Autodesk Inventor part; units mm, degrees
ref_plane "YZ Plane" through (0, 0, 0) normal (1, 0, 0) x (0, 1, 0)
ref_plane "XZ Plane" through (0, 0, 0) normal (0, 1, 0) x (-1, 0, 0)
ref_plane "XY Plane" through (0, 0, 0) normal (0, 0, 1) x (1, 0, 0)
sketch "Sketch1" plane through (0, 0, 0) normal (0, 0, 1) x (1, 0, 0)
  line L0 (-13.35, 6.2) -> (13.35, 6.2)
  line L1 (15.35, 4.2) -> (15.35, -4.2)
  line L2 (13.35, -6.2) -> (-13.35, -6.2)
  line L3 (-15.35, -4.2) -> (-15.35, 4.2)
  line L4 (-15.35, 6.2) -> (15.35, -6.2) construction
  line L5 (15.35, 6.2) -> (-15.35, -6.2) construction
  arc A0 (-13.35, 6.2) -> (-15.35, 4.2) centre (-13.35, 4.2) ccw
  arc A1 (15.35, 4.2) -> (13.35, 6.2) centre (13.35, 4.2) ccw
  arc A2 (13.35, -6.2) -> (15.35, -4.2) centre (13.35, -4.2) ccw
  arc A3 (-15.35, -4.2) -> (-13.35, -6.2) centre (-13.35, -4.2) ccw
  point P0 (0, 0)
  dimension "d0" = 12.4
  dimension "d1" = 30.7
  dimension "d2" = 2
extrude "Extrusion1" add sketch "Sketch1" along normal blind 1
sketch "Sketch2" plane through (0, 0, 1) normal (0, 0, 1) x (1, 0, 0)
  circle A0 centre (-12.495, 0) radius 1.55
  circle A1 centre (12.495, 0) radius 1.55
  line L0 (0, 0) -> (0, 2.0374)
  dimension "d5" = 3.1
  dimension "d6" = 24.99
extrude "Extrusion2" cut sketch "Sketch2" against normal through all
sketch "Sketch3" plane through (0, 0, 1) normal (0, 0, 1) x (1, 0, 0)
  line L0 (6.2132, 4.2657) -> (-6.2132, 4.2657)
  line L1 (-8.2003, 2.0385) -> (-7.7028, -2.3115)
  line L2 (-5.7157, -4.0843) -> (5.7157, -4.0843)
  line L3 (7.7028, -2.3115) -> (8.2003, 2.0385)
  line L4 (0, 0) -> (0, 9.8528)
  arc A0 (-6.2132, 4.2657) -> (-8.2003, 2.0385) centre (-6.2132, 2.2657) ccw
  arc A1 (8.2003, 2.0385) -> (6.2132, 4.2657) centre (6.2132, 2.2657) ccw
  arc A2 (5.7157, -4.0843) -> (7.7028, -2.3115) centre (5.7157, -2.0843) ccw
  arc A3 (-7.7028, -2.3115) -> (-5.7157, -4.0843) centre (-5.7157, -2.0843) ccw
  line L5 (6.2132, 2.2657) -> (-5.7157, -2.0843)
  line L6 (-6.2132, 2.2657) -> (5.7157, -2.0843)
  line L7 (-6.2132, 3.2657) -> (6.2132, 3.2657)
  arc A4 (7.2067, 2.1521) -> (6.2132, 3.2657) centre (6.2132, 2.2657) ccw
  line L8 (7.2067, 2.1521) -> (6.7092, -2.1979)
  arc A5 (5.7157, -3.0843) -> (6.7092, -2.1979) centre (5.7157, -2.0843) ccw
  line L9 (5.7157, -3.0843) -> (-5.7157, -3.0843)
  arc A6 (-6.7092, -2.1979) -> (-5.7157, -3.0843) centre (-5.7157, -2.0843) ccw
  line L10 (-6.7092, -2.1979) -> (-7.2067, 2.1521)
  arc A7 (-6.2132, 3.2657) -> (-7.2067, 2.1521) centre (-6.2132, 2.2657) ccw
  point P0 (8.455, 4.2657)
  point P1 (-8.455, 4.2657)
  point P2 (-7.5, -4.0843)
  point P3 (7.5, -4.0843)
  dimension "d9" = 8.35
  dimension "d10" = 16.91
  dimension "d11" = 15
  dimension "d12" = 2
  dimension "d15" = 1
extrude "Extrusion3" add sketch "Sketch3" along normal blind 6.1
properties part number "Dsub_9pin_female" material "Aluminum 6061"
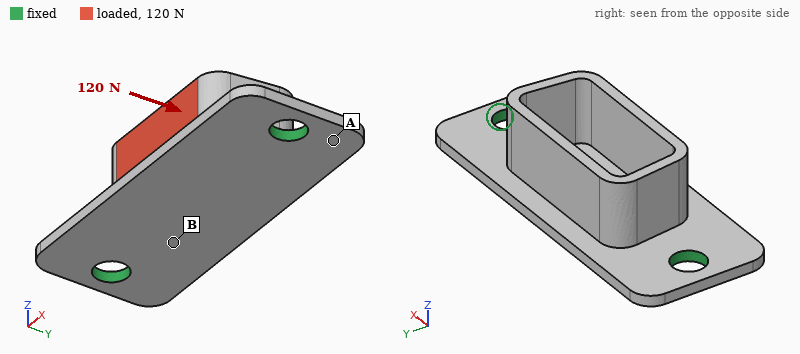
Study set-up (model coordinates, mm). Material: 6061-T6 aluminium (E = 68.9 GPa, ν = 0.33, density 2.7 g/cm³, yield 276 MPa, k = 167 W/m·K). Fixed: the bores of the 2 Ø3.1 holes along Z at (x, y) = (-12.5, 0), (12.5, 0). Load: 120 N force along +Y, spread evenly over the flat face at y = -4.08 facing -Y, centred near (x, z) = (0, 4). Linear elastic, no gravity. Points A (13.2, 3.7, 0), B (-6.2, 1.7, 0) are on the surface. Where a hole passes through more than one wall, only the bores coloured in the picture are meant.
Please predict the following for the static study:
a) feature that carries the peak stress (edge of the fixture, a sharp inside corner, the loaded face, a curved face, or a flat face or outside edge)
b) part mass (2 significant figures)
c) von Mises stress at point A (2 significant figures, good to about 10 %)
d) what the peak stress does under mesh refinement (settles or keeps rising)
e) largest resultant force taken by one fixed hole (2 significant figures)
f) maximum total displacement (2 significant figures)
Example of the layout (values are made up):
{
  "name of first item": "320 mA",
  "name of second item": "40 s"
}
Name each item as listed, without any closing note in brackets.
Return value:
{
  "feature that carries the peak stress": "edge of the fixture",
  "part mass": "1.7 g",
  "von Mises stress at point A": "38 MPa",
  "what the peak stress does under mesh refinement": "keeps rising",
  "largest resultant force taken by one fixed hole": "60 N",
  "maximum total displacement": "75 µm"
}
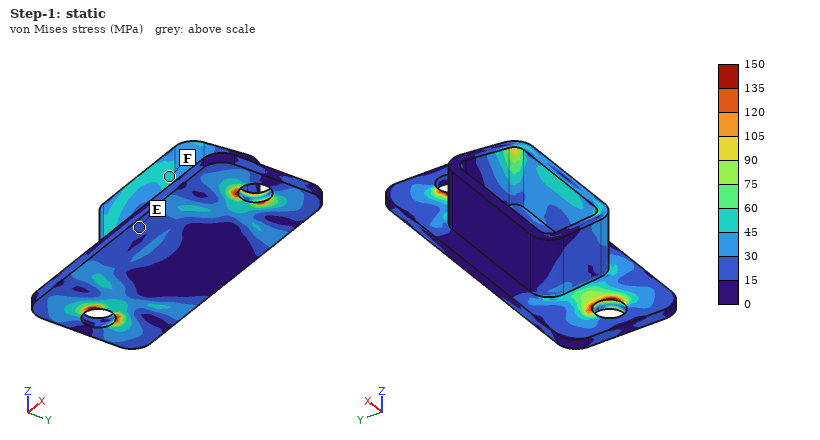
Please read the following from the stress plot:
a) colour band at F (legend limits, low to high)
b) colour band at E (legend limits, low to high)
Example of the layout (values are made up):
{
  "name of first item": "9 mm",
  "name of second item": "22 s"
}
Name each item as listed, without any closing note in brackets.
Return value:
{
  "colour band at F": "45 to 60 MPa",
  "colour band at E": "15 to 30 MPa"
}
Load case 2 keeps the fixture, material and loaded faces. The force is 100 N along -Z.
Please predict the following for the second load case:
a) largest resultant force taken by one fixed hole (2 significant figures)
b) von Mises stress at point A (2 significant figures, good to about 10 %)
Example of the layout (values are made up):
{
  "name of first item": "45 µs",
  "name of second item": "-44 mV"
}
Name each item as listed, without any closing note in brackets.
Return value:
{
  "largest resultant force taken by one fixed hole": "58 N",
  "von Mises stress at point A": "25 MPa"
}
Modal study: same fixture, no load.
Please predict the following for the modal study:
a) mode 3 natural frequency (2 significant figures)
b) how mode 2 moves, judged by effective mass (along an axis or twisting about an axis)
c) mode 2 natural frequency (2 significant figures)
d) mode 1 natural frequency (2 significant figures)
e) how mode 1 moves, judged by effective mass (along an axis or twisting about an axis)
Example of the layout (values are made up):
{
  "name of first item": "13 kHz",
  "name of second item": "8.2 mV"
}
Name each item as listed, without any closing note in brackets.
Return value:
{
  "mode 3 natural frequency": "20 kHz",
  "how mode 2 moves, judged by effective mass": "along Z",
  "mode 2 natural frequency": "15 kHz",
  "mode 1 natural frequency": "8400 Hz",
  "how mode 1 moves, judged by effective mass": "along Y"
}
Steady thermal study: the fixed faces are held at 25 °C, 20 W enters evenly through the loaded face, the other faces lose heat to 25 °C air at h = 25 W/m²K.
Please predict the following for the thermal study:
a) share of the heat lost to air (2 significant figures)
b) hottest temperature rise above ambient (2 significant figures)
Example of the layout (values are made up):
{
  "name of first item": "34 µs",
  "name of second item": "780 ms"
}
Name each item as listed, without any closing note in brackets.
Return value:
{
  "share of the heat lost to air": "4.0 %",
  "hottest temperature rise above ambient": "64 K"
}
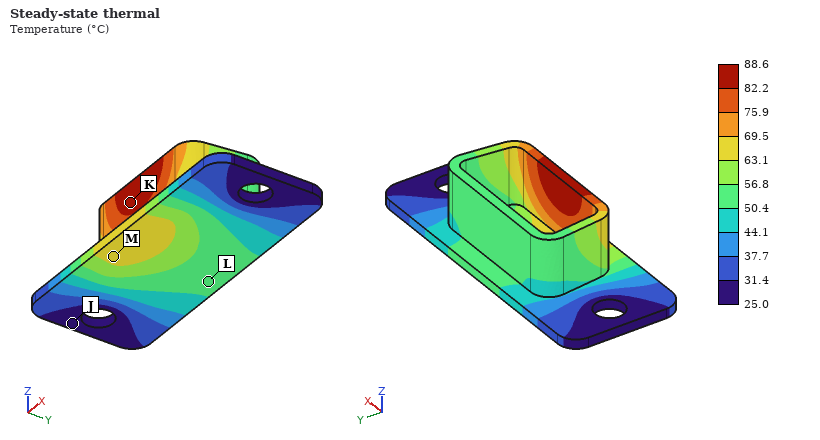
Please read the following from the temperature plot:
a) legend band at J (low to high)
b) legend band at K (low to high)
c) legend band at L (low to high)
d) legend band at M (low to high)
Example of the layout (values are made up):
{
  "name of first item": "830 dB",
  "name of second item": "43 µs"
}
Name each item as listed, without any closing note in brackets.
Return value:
{
  "legend band at J": "25.0 to 31.4 °C",
  "legend band at K": "82.2 to 88.6 °C",
  "legend band at L": "50.4 to 56.8 °C",
  "legend band at M": "63.1 to 69.5 °C"
}
